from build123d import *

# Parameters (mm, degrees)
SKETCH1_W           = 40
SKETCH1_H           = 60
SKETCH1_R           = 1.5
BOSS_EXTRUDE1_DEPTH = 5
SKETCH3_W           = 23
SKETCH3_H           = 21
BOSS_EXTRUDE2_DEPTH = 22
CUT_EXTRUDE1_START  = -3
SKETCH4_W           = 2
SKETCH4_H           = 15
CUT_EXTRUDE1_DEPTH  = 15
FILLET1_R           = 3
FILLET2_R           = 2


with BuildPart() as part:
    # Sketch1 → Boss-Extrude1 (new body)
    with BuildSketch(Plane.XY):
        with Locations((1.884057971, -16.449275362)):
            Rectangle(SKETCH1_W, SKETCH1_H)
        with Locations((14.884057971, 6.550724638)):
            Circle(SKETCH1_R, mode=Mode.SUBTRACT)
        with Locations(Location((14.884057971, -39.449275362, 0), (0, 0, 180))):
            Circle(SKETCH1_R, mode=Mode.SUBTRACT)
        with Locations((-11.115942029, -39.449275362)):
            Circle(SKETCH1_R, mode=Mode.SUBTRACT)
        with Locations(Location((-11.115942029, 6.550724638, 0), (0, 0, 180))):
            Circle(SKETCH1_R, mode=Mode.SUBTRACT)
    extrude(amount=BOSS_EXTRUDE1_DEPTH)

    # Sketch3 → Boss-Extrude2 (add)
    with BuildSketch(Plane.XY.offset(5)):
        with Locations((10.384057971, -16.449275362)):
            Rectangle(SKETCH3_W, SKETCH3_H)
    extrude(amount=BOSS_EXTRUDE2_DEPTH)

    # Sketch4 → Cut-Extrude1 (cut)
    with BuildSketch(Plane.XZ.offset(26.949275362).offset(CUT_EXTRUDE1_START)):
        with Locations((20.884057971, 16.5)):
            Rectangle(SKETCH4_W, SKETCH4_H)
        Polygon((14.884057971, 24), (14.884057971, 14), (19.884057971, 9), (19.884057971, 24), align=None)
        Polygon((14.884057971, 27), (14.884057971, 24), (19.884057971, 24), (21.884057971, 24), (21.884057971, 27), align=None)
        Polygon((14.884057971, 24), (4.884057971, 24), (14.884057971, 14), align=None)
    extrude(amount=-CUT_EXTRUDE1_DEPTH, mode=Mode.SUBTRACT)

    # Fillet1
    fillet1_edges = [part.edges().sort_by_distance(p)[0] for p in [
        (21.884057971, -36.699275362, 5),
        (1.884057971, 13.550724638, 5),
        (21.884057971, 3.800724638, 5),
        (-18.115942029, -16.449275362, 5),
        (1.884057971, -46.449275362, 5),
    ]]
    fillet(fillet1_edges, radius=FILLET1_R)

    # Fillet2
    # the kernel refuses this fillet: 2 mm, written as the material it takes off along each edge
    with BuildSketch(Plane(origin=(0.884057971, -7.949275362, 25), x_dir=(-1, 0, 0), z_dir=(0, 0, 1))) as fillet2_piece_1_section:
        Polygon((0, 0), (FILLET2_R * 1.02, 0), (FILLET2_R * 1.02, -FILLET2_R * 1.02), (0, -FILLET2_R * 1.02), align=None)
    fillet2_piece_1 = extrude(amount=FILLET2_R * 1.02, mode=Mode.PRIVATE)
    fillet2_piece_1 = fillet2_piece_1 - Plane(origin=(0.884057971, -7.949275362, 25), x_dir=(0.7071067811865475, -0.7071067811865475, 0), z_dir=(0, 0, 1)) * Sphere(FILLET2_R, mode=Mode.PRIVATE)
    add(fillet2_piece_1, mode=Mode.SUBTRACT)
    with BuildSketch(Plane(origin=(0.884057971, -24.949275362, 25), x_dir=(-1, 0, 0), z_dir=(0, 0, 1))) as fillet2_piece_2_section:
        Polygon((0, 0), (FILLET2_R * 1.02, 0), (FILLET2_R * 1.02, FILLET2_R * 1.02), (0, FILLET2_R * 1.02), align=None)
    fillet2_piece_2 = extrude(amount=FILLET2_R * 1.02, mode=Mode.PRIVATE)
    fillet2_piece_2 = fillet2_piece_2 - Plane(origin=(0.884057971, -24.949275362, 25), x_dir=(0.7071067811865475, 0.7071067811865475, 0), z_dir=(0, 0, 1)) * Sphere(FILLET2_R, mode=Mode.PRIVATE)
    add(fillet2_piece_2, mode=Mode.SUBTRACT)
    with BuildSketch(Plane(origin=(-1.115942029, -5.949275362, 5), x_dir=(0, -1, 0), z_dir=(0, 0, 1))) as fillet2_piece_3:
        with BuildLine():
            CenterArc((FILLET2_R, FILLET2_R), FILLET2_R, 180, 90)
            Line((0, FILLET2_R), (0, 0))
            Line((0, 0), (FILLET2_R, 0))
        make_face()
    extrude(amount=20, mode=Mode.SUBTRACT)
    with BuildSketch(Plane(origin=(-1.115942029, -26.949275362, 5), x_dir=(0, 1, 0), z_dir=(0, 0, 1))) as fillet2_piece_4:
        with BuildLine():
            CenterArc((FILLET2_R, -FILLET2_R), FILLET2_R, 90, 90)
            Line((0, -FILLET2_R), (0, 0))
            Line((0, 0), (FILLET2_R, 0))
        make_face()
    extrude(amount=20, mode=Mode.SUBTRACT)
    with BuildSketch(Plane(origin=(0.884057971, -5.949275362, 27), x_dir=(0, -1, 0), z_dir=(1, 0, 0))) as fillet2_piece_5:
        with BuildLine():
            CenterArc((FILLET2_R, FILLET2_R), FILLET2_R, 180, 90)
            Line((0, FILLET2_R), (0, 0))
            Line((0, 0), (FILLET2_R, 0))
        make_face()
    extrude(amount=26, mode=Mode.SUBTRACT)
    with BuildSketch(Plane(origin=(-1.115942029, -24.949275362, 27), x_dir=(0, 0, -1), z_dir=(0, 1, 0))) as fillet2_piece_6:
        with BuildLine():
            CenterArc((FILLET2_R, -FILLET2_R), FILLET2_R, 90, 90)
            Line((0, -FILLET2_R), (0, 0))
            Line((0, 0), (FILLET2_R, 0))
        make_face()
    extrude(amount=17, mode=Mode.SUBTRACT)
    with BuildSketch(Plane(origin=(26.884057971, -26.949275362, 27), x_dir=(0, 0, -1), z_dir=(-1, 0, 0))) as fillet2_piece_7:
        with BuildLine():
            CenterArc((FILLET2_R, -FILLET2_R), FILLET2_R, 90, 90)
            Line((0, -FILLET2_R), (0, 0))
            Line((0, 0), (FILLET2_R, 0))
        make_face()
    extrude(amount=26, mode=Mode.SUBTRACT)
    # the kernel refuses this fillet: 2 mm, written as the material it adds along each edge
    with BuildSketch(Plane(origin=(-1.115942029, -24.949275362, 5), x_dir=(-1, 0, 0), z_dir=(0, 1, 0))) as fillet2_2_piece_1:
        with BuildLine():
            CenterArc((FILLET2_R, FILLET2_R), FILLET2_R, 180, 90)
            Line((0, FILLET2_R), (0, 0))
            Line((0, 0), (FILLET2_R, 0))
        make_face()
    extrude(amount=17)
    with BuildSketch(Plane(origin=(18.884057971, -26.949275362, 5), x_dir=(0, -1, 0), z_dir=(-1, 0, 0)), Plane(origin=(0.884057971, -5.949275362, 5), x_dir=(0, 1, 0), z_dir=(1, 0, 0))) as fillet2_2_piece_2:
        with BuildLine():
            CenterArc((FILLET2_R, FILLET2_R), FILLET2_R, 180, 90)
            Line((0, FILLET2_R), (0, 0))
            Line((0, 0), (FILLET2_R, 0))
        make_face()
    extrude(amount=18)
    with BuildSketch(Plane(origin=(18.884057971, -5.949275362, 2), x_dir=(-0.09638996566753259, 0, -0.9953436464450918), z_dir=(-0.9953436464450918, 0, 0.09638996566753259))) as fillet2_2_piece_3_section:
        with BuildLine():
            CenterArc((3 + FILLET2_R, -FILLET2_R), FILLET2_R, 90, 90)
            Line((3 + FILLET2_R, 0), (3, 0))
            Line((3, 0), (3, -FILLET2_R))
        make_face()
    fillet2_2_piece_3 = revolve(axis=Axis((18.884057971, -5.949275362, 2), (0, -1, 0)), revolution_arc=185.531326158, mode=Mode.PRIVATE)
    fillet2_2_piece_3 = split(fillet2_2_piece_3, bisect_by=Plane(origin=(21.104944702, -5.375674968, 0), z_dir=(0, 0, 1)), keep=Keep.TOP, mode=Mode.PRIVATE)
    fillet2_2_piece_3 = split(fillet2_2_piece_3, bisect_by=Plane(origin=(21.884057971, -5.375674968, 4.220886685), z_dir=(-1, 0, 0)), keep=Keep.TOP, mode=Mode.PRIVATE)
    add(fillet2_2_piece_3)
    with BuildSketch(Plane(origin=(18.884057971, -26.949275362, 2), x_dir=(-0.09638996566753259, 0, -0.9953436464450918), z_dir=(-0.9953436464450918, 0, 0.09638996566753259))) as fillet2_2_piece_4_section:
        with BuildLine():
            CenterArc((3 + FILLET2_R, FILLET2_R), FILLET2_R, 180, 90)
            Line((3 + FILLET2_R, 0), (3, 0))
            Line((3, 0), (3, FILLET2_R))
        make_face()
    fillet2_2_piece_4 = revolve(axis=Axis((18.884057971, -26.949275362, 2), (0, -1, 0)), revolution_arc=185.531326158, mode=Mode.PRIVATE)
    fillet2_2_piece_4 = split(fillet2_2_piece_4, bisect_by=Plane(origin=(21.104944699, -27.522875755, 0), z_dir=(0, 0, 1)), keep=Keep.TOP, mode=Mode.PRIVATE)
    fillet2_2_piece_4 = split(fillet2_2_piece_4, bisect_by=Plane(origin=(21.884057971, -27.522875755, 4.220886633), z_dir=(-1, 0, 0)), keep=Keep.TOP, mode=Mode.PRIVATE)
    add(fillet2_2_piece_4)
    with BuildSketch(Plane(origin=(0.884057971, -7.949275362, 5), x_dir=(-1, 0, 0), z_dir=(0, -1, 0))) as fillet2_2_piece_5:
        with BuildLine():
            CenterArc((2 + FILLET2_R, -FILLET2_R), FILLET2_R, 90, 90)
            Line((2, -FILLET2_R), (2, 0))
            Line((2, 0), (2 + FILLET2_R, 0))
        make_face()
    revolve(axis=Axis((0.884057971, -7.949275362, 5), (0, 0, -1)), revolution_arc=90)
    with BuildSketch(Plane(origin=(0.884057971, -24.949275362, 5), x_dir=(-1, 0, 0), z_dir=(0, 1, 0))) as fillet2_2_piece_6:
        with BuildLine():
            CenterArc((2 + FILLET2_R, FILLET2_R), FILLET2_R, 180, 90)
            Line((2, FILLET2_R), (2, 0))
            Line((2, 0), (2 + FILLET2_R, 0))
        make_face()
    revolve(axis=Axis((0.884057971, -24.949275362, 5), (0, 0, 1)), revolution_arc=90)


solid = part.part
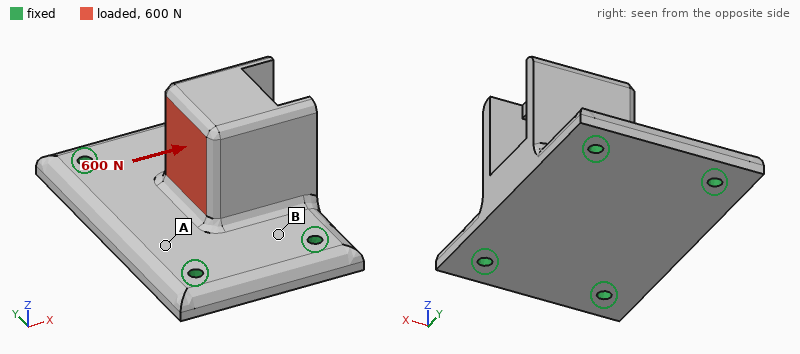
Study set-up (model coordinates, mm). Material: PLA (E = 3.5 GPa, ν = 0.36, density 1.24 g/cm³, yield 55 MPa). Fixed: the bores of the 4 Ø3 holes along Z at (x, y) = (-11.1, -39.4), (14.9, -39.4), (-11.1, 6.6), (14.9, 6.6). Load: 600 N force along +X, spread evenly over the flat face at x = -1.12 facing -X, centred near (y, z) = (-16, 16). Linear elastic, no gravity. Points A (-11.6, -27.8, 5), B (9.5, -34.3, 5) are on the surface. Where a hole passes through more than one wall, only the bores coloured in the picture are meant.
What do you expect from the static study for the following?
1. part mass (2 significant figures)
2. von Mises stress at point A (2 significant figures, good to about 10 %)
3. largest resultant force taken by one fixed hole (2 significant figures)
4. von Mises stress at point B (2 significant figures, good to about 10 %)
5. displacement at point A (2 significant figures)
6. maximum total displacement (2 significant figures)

24 g
4.7 MPa
250 N
12 MPa
0.091 mm
0.40 mm
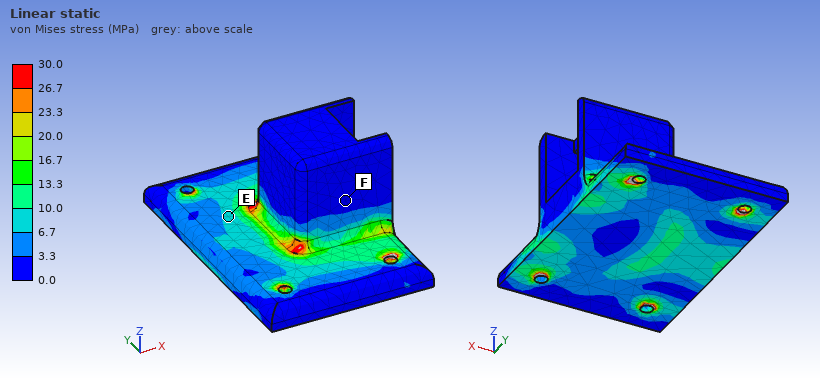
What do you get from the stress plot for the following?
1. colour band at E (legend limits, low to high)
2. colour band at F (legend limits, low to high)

6.7 to 10.0 MPa
0.0 to 3.3 MPa
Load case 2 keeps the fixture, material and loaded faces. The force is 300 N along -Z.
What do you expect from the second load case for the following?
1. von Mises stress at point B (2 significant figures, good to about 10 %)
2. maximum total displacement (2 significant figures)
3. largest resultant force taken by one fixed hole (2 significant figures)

1.7 MPa
0.14 mm
93 N
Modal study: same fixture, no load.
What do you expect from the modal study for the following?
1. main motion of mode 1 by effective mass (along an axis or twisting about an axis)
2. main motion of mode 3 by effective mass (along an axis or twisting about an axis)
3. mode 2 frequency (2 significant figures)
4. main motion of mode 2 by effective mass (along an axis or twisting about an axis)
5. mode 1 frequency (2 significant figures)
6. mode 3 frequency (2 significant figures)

along X
along Y
2800 Hz
along Z
2300 Hz
3400 Hz
